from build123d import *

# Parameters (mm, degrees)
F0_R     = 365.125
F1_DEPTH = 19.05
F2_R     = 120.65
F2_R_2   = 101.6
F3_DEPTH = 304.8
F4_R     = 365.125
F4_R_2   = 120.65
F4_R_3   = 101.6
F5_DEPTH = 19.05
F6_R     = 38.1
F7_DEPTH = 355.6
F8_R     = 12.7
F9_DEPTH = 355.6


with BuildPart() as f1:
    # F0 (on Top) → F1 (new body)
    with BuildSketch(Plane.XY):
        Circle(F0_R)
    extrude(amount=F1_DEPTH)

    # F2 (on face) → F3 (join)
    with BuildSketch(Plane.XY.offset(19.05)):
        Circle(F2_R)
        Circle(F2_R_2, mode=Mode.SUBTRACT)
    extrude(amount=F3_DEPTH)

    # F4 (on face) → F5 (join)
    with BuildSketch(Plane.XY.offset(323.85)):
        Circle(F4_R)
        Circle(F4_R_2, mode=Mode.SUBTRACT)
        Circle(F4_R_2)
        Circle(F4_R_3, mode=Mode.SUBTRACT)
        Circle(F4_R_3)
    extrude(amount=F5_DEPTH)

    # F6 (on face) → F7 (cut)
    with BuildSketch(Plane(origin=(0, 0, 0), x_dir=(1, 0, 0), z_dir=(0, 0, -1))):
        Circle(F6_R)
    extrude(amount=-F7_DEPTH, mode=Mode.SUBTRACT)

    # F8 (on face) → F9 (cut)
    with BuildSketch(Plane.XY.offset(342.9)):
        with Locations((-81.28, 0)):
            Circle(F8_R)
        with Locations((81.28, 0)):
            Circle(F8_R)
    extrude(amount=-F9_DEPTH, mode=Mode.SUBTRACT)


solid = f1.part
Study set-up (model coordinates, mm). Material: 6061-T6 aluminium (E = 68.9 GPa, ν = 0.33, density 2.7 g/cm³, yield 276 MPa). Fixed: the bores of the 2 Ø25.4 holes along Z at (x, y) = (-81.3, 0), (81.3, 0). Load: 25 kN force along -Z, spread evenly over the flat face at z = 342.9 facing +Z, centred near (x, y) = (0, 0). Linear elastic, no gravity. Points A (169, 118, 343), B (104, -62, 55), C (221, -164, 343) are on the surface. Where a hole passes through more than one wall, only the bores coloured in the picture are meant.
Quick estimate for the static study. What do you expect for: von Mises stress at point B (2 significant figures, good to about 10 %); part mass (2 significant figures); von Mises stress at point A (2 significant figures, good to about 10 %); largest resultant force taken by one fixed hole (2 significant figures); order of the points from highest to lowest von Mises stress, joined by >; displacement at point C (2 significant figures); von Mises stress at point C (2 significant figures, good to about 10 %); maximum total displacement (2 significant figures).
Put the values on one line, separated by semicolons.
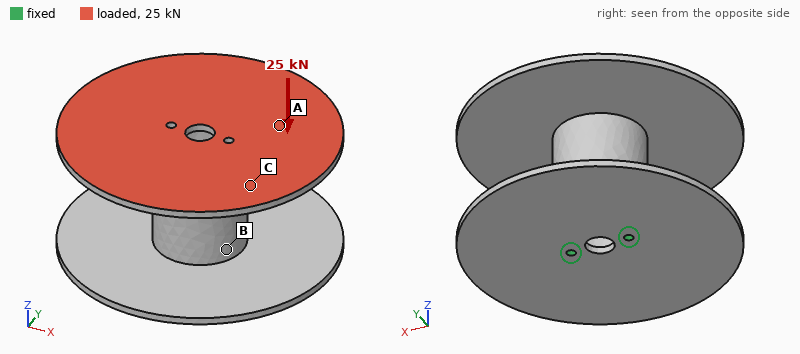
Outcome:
3.1 MPa; 53 kg; 14 MPa; 13 kN; A > C > B; 0.53 mm; 9.5 MPa; 0.87 mm
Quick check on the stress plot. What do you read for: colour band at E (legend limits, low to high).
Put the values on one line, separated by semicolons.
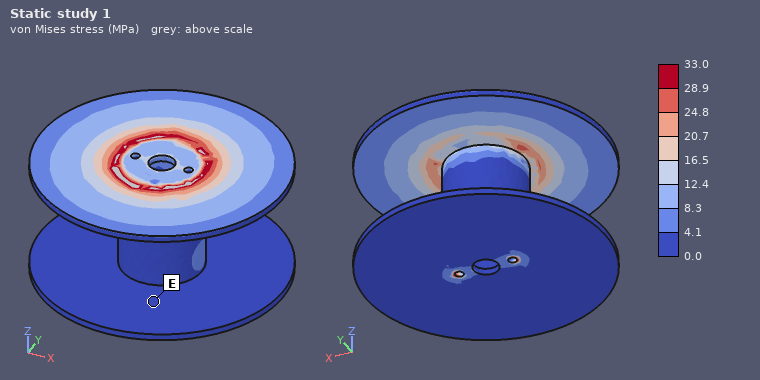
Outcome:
0.0 to 4.1 MPa
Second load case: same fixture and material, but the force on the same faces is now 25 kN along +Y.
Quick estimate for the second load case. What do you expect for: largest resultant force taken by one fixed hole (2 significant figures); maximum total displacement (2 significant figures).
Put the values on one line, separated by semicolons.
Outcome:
13 kN; 4.5 mm
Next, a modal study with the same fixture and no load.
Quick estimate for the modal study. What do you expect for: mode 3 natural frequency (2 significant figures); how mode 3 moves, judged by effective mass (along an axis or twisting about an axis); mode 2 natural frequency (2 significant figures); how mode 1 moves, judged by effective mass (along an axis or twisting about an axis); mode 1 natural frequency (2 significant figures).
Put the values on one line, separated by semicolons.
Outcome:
210 Hz; along Z; 180 Hz; along Y; 74 Hz
